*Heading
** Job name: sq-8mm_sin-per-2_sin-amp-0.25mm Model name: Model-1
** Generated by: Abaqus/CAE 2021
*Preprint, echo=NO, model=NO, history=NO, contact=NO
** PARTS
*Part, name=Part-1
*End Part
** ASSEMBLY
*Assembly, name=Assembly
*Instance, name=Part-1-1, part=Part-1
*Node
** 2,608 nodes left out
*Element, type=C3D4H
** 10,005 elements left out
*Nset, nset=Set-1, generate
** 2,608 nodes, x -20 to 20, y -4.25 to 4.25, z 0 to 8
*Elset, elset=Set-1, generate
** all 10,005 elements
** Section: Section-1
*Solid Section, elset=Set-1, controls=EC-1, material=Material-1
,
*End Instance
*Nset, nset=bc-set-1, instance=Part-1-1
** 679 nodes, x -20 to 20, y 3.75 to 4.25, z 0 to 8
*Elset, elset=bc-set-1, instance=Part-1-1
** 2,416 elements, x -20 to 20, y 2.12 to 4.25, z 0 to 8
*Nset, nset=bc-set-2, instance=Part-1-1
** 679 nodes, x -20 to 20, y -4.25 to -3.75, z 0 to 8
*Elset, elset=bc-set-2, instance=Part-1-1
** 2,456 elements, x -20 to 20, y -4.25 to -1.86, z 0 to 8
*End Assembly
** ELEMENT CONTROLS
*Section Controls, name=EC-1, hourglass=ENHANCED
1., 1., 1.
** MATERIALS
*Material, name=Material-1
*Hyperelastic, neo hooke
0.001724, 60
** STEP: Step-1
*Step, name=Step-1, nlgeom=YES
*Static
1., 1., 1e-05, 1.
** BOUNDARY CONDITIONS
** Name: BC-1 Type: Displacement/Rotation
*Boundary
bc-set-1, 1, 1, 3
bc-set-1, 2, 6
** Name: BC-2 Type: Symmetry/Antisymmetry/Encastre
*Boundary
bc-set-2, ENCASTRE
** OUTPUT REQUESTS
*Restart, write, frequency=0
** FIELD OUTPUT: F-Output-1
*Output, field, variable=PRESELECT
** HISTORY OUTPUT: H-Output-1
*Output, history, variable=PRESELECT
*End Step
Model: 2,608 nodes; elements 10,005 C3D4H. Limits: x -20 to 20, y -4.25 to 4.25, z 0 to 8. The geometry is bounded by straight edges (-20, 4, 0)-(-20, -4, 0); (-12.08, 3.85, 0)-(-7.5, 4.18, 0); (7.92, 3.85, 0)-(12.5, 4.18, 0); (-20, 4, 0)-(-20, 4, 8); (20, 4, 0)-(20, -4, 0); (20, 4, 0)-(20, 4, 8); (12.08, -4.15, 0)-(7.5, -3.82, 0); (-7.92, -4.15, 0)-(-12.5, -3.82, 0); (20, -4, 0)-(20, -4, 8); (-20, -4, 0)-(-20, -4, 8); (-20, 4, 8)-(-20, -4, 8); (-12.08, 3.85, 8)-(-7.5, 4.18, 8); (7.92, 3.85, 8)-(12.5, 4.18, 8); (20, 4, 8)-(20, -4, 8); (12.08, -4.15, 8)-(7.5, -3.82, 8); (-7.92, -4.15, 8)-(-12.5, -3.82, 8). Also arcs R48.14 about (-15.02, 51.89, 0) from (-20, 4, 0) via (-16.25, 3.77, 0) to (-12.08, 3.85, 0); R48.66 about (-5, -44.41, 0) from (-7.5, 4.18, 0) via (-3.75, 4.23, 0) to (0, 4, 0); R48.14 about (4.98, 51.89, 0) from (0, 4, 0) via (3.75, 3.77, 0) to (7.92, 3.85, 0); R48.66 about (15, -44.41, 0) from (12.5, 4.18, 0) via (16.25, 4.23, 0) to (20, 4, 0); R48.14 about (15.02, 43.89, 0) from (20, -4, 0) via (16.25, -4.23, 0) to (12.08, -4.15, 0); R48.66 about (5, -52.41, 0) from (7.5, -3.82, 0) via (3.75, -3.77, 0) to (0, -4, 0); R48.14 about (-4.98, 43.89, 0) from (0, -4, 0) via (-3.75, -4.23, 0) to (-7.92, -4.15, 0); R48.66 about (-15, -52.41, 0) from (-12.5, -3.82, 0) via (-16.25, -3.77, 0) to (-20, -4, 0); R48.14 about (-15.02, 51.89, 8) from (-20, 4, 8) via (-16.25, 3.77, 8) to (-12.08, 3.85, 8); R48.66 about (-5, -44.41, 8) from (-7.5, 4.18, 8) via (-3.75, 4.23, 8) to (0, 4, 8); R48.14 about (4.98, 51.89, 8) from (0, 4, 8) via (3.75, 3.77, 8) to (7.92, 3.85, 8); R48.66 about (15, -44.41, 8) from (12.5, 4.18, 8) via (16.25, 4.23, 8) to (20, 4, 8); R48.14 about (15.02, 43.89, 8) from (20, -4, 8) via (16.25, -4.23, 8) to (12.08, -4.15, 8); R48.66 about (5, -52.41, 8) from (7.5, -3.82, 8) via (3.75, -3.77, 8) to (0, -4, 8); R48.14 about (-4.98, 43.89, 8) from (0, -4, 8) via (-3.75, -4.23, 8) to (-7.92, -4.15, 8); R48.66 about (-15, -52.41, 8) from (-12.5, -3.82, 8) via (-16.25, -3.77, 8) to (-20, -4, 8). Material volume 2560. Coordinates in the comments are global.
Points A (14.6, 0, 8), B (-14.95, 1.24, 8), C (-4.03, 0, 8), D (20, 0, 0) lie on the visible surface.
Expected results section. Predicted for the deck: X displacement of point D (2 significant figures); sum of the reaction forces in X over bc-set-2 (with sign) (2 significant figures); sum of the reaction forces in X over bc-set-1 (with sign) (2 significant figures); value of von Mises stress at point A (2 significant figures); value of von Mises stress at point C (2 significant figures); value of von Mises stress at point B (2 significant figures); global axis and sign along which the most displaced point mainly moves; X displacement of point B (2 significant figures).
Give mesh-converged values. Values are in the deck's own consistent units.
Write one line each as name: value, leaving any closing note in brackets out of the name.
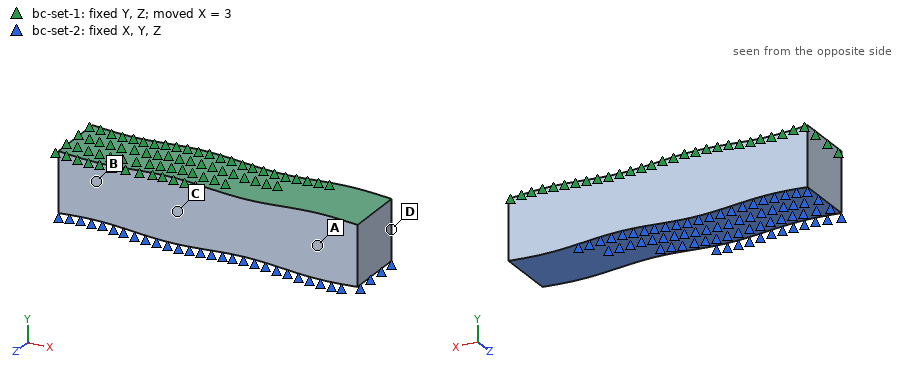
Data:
X displacement of point D: 1.5
sum of the reaction forces in X over bc-set-2 (with sign): -0.39
sum of the reaction forces in X over bc-set-1 (with sign): 0.39
value of von Mises stress at point A: 0.0024
value of von Mises stress at point C: 0.0023
value of von Mises stress at point B: 0.0025
global axis and sign along which the most displaced point mainly moves: +X
X displacement of point B: 2.0
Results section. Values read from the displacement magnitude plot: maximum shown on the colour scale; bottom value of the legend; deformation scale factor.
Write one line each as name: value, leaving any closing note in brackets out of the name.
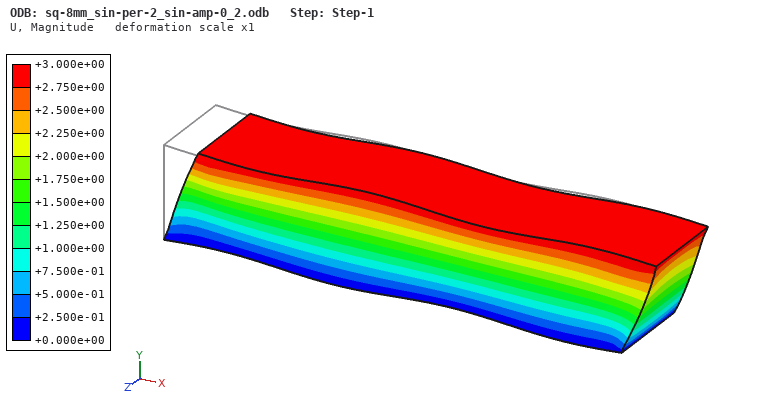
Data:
maximum shown on the colour scale: +3.000e+00
bottom value of the legend: +0.000e+00
deformation scale factor: 1
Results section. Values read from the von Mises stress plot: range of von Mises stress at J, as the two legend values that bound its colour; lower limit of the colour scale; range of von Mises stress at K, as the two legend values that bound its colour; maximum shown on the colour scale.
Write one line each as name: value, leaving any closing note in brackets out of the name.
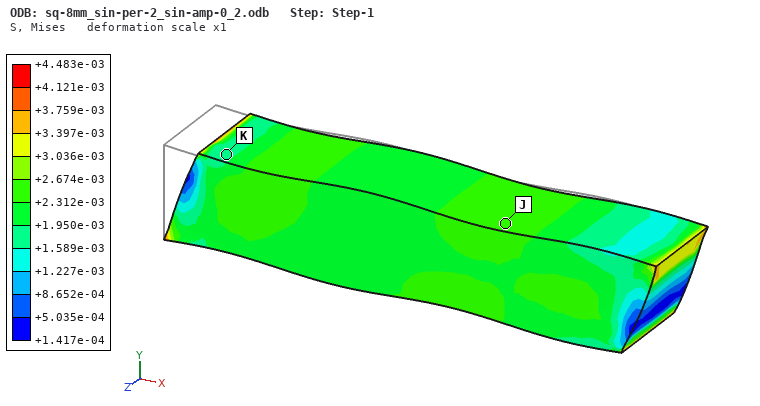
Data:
range of von Mises stress at J, as the two legend values that bound its colour: +2.312e-03 to +2.674e-03
lower limit of the colour scale: +1.417e-04
range of von Mises stress at K, as the two legend values that bound its colour: +1.589e-03 to +1.950e-03
maximum shown on the colour scale: +4.483e-03
